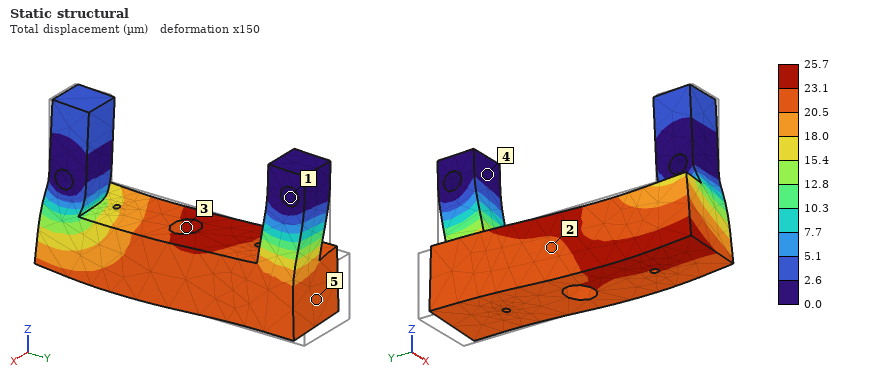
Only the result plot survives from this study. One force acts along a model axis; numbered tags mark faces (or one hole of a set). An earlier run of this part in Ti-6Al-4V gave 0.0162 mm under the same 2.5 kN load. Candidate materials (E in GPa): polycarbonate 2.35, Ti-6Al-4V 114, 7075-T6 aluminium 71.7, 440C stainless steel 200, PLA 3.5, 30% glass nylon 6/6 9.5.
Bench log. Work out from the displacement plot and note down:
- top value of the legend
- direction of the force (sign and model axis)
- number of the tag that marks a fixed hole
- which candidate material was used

25.7 µm
-Y
1
7075-T6 aluminium
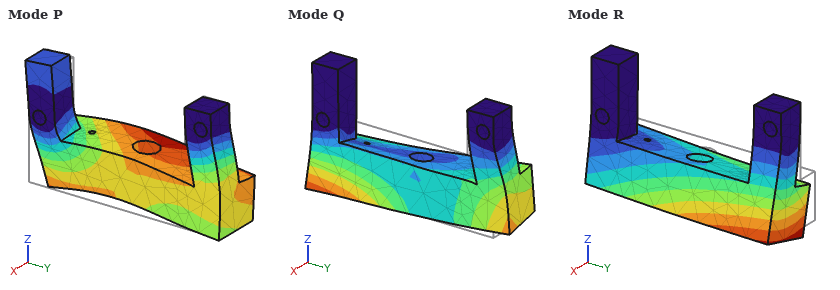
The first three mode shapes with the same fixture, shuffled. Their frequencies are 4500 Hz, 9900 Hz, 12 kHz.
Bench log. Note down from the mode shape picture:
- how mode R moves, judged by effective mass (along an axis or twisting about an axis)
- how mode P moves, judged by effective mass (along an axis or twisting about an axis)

along X
along Y
